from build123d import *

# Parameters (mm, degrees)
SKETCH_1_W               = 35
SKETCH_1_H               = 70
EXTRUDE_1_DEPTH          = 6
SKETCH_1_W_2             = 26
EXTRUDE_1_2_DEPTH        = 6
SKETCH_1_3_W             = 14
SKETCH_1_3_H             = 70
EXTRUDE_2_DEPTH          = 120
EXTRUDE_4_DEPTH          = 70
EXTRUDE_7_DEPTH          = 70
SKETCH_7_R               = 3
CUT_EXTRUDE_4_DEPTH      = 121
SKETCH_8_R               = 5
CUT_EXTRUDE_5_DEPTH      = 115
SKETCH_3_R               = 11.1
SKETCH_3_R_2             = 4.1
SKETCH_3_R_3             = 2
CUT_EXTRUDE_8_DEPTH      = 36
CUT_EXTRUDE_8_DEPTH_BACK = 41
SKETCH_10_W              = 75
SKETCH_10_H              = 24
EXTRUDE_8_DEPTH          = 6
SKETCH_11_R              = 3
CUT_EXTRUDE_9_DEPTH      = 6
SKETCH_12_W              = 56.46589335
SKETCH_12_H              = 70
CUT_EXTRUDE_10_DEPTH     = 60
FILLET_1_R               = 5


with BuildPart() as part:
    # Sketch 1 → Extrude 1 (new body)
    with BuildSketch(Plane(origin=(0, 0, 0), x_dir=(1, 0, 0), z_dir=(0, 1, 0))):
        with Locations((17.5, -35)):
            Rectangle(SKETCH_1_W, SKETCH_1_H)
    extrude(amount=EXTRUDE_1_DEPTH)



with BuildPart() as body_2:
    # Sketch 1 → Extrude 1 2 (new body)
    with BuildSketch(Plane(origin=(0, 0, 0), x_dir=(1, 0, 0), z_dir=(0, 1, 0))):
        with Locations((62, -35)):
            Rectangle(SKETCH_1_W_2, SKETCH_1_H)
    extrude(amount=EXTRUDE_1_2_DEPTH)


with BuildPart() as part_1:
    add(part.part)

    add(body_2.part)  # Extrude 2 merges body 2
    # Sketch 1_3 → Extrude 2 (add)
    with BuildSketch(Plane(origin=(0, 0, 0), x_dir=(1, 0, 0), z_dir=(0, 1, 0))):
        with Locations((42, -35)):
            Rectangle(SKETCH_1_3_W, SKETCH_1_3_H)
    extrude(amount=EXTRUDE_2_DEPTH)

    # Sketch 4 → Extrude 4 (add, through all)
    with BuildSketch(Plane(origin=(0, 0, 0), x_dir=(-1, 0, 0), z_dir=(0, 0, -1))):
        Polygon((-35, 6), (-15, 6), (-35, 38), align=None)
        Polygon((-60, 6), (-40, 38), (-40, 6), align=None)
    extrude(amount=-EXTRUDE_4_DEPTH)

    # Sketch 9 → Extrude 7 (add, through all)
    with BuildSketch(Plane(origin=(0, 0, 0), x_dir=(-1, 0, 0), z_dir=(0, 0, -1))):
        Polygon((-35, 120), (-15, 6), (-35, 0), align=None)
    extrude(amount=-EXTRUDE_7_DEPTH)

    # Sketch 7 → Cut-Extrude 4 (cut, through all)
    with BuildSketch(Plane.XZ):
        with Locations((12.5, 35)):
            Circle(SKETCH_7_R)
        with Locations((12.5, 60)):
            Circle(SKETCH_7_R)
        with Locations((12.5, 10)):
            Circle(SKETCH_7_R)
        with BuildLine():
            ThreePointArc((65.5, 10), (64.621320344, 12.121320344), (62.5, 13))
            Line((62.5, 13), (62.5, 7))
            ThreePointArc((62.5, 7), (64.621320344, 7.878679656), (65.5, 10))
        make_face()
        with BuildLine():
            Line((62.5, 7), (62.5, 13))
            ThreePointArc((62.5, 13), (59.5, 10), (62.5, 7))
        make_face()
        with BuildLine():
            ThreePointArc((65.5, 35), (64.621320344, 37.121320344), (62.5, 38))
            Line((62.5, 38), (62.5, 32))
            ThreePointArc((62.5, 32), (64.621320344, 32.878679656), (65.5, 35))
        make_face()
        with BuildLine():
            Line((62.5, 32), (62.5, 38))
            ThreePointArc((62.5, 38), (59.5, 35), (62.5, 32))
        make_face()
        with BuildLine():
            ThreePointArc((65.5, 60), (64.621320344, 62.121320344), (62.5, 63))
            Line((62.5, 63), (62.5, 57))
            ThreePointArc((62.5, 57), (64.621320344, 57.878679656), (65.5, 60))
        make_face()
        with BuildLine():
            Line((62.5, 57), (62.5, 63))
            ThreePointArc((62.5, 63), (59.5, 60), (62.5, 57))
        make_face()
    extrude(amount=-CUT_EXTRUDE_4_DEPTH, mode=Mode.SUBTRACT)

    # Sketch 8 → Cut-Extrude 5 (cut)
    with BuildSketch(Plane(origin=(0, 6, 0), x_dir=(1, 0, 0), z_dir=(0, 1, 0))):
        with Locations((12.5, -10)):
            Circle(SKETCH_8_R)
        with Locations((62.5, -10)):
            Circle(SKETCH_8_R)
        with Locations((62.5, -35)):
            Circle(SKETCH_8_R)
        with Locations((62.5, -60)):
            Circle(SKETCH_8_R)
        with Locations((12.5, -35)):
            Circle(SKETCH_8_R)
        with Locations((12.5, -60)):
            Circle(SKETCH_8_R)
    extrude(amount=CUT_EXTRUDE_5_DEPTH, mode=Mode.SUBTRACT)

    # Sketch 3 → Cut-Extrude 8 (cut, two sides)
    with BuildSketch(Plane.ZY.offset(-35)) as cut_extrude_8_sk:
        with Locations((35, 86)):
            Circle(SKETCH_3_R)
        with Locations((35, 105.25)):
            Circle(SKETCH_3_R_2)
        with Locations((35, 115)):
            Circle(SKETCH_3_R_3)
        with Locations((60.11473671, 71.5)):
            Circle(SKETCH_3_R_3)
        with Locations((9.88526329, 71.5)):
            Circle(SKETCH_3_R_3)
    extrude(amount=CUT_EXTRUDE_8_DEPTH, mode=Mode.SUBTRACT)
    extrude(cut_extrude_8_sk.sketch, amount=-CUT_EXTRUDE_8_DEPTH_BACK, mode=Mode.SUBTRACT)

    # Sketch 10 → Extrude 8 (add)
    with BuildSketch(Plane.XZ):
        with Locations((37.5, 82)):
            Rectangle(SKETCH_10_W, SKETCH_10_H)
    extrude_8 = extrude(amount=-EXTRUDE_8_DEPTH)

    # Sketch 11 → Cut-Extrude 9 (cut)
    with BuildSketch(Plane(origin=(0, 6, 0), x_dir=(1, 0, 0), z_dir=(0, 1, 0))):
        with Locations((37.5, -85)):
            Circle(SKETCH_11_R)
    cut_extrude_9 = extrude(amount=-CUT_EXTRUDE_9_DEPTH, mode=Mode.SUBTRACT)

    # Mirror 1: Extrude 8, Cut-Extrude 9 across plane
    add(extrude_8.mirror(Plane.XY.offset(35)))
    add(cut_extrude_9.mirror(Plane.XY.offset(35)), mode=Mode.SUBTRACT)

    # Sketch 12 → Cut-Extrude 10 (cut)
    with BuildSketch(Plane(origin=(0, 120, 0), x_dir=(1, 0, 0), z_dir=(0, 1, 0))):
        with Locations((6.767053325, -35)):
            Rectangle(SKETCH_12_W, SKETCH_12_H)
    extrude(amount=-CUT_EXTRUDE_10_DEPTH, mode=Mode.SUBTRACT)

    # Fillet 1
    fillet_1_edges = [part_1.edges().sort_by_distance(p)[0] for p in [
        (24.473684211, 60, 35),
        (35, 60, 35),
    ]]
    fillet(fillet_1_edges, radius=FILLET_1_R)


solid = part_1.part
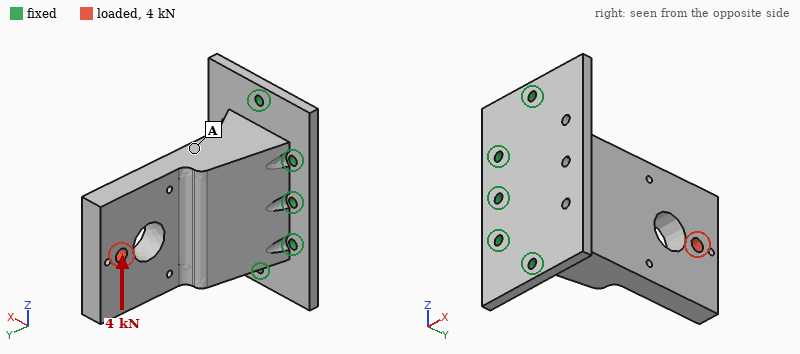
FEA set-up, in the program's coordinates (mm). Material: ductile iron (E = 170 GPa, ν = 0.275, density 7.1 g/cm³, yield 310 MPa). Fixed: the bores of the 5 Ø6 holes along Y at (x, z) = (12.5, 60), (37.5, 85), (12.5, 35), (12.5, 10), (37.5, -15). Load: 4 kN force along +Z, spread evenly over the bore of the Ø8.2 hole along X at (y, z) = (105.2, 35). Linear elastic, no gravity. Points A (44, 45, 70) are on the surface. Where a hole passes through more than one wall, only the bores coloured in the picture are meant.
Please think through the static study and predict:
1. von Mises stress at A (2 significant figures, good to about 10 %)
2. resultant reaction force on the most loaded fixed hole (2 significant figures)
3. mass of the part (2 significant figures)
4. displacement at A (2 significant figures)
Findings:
15 MPa
5.0 kN
1.6 kg
19 µm
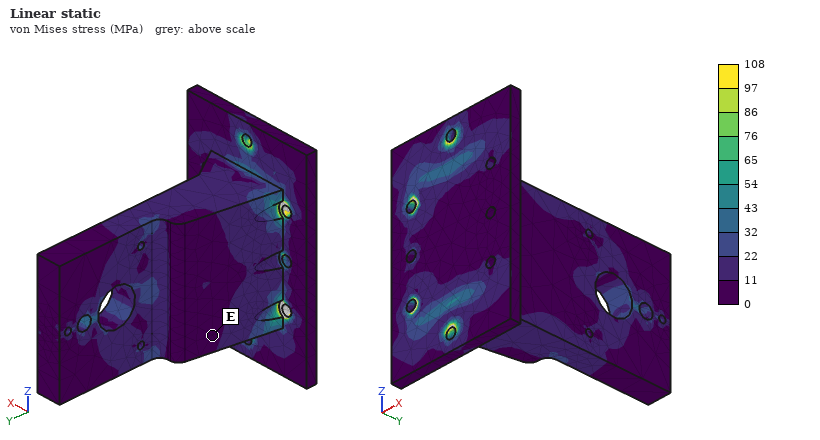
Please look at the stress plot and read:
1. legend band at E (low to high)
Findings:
0 to 11 MPa
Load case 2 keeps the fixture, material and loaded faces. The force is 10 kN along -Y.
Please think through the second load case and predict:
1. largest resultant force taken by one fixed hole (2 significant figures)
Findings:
4.5 kN
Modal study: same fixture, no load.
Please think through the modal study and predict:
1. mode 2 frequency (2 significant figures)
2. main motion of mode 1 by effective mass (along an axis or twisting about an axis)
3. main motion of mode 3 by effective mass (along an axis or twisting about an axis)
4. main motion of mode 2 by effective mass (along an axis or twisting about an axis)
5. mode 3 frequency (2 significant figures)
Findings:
2500 Hz
along X
along Y
along Z
3400 Hz
